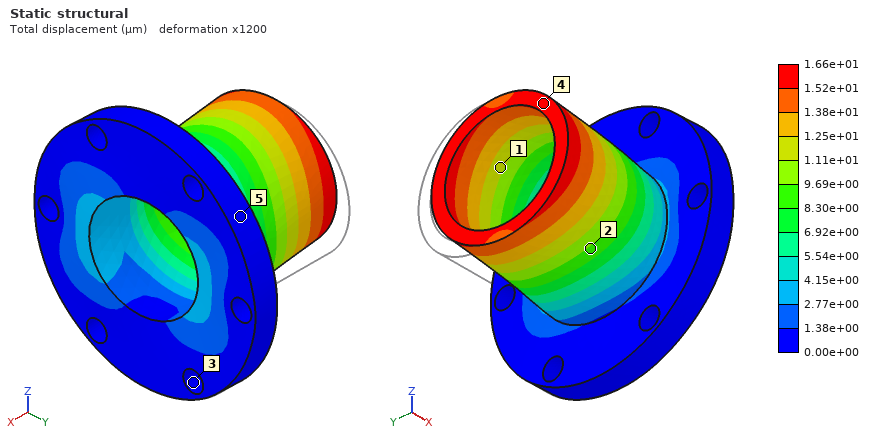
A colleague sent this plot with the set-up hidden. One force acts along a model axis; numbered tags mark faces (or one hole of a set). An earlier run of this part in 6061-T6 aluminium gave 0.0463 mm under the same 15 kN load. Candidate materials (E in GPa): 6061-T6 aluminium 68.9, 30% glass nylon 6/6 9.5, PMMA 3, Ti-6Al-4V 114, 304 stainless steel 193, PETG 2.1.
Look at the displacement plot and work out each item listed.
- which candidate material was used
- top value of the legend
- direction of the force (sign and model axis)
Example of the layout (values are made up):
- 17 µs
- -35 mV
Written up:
- 304 stainless steel
- 1.66e+01 µm
- -Y
